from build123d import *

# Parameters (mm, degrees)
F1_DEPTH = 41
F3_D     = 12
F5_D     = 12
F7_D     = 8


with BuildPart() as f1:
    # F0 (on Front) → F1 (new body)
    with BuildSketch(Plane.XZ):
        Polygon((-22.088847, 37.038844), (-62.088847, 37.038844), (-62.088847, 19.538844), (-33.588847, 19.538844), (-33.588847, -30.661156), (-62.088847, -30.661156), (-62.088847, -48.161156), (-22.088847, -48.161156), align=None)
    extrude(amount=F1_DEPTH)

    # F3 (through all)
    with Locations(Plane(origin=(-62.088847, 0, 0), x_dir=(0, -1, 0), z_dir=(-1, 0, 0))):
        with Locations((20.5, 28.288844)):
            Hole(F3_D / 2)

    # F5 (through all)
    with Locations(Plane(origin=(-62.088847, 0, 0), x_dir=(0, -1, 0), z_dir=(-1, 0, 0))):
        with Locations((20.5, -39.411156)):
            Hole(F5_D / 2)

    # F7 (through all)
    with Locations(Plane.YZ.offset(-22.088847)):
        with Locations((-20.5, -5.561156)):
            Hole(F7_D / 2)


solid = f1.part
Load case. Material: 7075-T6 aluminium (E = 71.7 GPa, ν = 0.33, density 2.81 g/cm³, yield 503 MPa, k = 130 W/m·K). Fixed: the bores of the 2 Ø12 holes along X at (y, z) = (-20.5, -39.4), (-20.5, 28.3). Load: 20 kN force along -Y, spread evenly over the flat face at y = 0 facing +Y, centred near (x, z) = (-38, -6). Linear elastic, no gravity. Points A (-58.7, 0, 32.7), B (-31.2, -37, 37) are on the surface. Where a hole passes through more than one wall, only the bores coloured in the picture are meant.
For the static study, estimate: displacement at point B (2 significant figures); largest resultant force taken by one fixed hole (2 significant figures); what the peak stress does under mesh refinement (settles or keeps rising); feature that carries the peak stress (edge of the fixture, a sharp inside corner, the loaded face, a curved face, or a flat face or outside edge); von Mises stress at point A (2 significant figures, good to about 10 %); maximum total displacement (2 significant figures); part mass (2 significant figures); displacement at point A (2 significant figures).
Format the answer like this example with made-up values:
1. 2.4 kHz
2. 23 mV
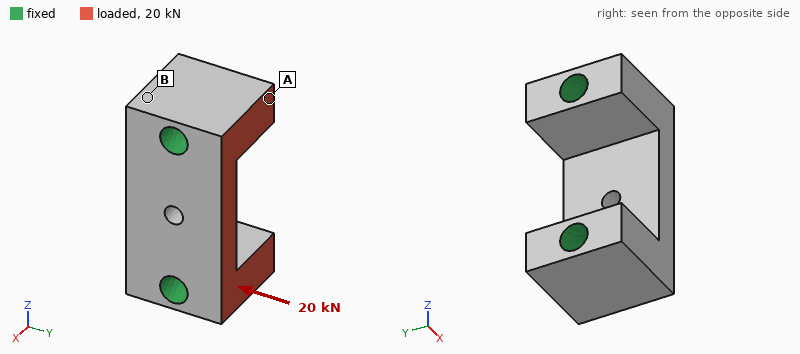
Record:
1. 1.5 µm
2. 10 kN
3. keeps rising
4. edge of the fixture
5. 10 MPa
6. 9.2 µm
7. 200 g
8. 2.3 µm
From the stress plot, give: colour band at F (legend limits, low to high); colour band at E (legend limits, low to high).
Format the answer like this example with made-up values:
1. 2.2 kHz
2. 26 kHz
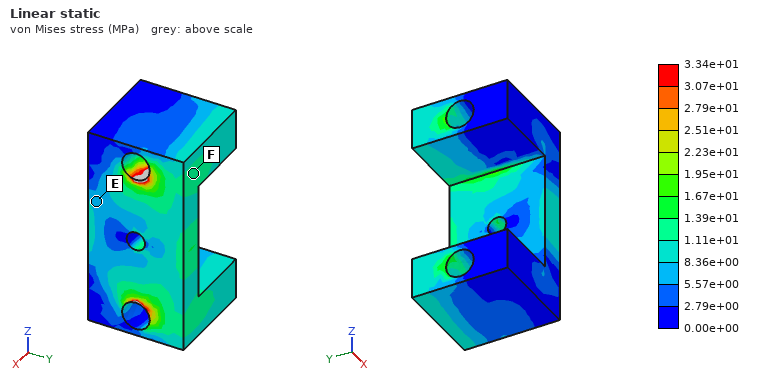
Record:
1. 1.11e+01 to 1.39e+01 MPa
2. 5.57e+00 to 8.36e+00 MPa
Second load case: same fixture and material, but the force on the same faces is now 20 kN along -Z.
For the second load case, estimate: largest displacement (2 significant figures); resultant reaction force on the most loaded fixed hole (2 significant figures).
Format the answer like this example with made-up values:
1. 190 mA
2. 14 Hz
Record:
1. 20 µm
2. 10 kN
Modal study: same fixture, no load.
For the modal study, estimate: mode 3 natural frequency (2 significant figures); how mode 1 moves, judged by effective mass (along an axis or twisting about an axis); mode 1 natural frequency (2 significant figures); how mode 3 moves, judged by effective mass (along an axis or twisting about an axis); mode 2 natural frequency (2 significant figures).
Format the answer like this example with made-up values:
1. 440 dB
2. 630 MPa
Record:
1. 19 kHz
2. along X
3. 14 kHz
4. along Y
5. 17 kHz
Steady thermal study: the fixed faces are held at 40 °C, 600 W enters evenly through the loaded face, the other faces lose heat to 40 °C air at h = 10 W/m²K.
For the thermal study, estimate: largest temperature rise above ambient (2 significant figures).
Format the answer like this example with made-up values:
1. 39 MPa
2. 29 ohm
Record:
1. 66 K
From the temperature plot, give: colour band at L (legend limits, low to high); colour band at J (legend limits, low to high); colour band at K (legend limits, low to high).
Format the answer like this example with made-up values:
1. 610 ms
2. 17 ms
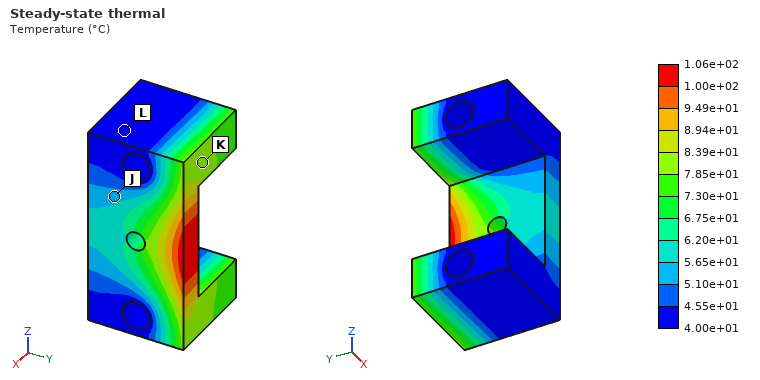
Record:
1. 4.00e+01 to 4.55e+01 °C
2. 5.10e+01 to 5.65e+01 °C
3. 7.85e+01 to 8.39e+01 °C
